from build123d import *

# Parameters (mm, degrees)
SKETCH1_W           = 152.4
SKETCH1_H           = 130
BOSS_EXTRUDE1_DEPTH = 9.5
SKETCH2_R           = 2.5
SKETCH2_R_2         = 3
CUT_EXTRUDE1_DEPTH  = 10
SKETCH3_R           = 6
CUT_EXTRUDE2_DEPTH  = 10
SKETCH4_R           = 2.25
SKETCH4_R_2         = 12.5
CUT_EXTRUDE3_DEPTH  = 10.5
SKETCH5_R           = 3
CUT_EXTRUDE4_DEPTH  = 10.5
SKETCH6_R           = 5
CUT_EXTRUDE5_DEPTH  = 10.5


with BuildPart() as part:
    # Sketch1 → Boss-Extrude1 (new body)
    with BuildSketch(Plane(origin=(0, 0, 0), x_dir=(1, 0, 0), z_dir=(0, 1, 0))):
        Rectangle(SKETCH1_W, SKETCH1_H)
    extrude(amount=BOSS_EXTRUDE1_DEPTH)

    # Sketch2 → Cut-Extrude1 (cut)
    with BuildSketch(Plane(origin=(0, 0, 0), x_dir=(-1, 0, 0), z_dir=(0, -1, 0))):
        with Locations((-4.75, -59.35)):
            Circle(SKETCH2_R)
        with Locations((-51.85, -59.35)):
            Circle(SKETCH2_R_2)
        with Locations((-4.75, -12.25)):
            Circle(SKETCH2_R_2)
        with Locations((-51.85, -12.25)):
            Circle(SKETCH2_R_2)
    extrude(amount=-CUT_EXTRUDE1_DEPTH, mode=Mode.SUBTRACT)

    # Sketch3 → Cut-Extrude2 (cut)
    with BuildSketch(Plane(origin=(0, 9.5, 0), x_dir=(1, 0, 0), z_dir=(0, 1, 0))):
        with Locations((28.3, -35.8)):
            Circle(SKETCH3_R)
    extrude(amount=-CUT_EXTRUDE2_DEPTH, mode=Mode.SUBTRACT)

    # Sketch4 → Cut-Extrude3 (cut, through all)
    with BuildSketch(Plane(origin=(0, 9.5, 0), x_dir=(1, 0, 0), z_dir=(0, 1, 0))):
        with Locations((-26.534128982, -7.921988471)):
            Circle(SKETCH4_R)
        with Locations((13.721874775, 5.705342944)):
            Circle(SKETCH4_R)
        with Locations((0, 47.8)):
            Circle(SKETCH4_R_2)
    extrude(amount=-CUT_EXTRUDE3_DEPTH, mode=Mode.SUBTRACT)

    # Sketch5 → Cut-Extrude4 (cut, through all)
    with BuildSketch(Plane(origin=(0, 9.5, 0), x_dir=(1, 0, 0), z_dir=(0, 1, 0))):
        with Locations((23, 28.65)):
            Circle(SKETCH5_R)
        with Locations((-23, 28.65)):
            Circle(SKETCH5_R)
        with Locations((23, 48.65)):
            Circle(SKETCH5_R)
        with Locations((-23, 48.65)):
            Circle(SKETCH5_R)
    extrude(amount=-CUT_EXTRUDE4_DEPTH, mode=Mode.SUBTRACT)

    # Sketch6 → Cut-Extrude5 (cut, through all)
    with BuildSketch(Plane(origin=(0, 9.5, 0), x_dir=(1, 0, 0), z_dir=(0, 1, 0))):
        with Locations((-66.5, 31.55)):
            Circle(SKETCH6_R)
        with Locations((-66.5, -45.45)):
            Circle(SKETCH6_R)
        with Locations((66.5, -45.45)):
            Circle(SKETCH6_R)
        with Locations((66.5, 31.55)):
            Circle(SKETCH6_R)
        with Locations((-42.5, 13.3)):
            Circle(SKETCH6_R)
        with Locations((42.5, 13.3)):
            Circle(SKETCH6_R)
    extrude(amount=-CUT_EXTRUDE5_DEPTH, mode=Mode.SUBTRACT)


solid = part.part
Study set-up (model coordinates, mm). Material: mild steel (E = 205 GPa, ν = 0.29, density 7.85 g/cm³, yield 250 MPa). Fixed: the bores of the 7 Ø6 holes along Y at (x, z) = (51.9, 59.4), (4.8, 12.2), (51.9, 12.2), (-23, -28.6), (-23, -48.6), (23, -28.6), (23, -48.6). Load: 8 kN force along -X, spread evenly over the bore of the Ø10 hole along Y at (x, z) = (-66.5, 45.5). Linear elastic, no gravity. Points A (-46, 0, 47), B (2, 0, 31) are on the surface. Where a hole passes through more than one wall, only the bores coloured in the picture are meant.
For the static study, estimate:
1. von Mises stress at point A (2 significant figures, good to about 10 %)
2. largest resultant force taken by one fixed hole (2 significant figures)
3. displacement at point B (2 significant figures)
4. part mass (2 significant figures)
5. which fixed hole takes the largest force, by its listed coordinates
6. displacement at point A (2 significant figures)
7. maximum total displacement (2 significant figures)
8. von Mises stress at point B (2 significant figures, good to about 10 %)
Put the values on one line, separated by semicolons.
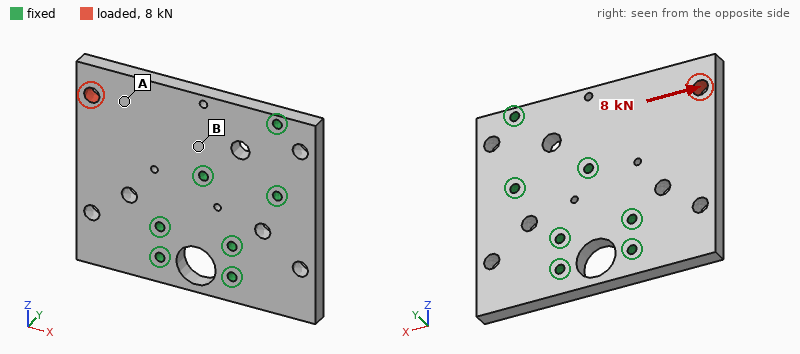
23 MPa; 4.1 kN; 2.3 µm; 1.4 kg; (4.8, 12.2); 7.8 µm; 14 µm; 11 MPa
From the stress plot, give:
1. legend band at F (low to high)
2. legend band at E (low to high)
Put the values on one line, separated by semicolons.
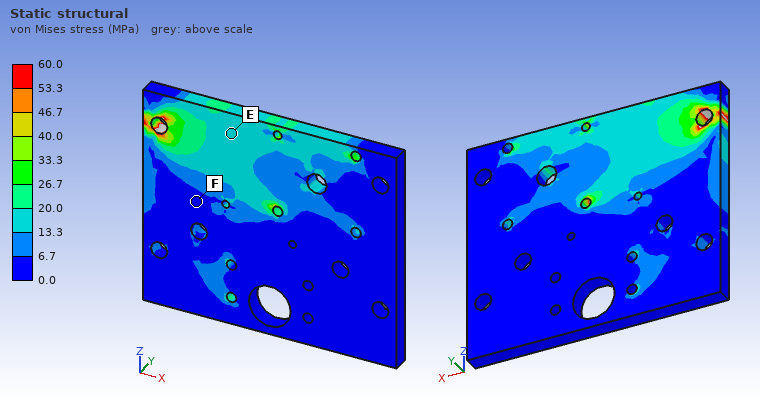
0.0 to 6.7 MPa; 13.3 to 20.0 MPa
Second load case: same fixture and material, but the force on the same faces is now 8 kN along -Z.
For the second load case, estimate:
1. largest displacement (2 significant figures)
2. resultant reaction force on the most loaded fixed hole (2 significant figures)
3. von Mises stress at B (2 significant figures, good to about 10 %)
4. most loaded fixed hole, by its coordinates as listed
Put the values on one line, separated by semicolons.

19 µm; 4.5 kN; 5.7 MPa; (-23, -28.6)
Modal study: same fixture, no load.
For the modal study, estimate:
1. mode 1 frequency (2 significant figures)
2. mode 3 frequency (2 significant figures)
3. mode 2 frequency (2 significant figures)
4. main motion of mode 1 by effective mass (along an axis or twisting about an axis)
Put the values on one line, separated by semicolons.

1300 Hz; 3700 Hz; 2900 Hz; along Y
